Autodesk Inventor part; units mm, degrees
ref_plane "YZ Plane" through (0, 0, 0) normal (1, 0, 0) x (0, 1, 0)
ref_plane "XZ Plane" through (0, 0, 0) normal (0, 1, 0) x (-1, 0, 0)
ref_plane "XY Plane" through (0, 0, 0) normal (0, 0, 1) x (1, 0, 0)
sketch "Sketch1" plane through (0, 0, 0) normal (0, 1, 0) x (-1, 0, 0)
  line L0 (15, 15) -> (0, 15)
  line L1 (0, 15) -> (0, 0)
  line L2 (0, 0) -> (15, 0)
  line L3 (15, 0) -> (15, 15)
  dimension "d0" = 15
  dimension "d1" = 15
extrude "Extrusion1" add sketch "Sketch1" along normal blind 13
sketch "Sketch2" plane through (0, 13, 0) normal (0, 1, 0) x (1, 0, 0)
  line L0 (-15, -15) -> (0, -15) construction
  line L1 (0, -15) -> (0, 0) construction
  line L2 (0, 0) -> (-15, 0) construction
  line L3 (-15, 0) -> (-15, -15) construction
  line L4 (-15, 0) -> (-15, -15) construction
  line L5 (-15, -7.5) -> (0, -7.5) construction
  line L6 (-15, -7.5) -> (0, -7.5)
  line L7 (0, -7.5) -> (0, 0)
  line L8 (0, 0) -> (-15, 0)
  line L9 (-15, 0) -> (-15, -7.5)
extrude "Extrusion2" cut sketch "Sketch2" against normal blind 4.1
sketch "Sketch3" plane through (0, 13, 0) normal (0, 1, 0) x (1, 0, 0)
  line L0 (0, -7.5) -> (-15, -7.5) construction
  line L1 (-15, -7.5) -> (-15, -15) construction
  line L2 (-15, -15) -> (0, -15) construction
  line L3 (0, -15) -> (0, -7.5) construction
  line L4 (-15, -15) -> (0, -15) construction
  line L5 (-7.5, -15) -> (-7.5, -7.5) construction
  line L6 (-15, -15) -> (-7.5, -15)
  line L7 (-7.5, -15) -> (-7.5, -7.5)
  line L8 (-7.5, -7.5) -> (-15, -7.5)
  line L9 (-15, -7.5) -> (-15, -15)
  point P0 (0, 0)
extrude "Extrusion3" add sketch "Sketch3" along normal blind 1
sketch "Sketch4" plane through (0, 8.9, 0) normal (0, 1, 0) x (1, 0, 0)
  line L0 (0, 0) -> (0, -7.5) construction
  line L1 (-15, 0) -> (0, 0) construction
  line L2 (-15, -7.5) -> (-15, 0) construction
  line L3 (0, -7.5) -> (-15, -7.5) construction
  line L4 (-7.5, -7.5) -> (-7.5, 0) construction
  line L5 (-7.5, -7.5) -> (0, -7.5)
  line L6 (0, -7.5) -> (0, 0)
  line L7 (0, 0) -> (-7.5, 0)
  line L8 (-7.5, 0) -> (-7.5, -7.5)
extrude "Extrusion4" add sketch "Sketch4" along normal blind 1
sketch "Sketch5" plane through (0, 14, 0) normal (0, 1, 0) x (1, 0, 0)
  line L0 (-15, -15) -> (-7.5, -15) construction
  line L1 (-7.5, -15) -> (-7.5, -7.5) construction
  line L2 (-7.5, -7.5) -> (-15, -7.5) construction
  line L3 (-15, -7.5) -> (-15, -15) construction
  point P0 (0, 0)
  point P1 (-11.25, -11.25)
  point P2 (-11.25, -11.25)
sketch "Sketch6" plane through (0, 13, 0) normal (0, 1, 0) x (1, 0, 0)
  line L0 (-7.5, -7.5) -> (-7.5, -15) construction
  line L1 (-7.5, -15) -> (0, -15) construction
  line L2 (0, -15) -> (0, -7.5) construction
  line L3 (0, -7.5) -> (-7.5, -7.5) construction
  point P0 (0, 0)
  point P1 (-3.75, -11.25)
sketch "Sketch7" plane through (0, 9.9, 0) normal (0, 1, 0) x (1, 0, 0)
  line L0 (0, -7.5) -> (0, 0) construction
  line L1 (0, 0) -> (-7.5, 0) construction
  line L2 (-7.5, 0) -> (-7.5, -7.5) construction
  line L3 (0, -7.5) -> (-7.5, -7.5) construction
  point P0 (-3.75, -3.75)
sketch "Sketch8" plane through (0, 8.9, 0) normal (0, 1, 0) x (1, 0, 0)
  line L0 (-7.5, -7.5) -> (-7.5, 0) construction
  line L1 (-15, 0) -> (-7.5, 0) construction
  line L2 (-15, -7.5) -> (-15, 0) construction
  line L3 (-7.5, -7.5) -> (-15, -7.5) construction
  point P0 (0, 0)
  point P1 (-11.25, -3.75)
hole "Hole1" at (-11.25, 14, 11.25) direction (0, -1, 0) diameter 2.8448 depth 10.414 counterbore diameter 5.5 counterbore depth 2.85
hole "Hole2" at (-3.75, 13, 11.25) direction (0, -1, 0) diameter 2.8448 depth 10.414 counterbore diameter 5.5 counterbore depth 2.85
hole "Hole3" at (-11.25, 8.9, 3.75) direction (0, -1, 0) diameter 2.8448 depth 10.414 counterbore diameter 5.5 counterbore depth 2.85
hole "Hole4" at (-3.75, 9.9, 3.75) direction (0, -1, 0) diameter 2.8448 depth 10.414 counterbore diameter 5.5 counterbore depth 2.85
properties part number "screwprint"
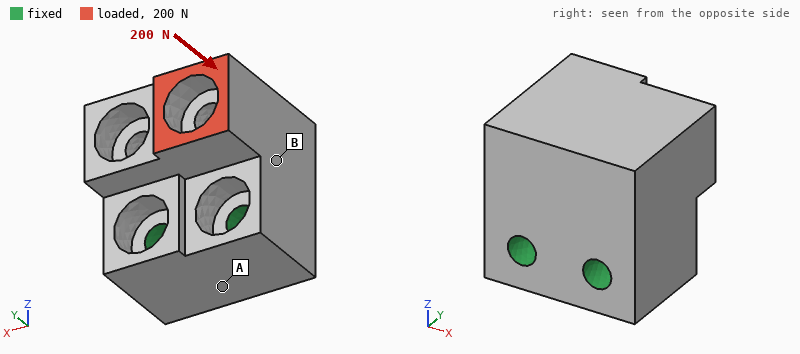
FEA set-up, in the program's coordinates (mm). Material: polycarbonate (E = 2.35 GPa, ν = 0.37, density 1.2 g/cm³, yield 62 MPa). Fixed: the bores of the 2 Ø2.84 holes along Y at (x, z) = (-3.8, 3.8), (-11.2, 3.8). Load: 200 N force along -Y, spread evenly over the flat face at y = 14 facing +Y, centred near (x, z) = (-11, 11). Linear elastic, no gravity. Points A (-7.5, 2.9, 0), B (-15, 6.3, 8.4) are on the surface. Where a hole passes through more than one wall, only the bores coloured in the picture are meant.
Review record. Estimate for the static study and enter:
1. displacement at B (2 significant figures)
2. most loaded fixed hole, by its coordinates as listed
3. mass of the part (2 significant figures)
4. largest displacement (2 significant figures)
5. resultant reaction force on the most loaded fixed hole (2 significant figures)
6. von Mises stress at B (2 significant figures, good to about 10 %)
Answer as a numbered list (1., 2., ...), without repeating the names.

1. 0.042 mm
2. (-11.2, 3.8)
3. 2.6 g
4. 0.13 mm
5. 150 N
6. 7.0 MPa
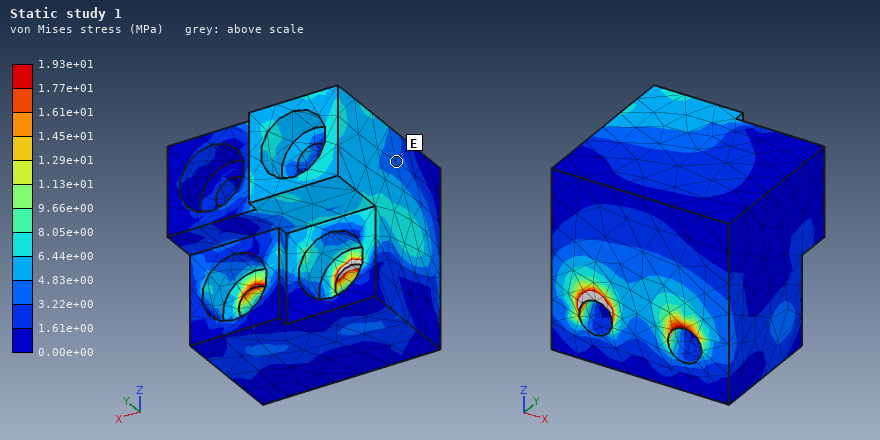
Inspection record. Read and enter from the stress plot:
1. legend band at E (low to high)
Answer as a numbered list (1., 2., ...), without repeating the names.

1. 3.22e+00 to 4.83e+00 MPa
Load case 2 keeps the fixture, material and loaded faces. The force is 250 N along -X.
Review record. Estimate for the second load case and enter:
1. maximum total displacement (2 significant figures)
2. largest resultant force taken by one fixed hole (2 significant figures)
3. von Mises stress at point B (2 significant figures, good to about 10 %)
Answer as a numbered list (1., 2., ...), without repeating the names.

1. 0.26 mm
2. 320 N
3. 12 MPa
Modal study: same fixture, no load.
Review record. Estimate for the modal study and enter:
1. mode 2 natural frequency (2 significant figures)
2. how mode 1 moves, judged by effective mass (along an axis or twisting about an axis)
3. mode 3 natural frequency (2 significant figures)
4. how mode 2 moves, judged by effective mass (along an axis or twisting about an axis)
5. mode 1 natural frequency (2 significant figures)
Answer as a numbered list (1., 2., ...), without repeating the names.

1. 10000 Hz
2. along Y
3. 12 kHz
4. along X
5. 7300 Hz
